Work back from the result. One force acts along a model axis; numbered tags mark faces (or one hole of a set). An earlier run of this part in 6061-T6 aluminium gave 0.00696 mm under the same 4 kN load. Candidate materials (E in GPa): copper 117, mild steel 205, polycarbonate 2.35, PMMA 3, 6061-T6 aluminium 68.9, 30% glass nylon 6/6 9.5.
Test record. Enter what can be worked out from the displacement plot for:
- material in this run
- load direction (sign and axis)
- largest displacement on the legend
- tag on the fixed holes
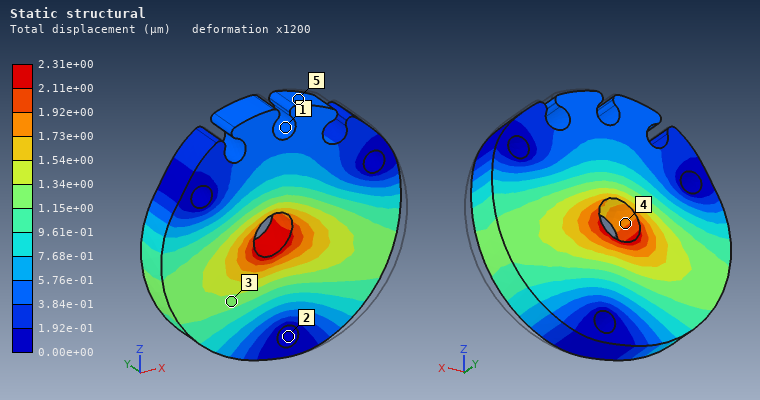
mild steel
-X
2.31e+00 µm
2
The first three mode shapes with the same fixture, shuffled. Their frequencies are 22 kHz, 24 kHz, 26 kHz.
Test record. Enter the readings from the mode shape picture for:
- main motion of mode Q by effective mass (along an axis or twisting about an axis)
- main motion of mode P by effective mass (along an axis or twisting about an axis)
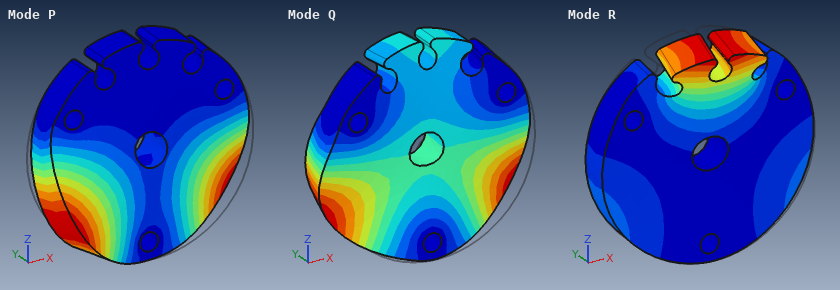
along Y
twisting about Z
